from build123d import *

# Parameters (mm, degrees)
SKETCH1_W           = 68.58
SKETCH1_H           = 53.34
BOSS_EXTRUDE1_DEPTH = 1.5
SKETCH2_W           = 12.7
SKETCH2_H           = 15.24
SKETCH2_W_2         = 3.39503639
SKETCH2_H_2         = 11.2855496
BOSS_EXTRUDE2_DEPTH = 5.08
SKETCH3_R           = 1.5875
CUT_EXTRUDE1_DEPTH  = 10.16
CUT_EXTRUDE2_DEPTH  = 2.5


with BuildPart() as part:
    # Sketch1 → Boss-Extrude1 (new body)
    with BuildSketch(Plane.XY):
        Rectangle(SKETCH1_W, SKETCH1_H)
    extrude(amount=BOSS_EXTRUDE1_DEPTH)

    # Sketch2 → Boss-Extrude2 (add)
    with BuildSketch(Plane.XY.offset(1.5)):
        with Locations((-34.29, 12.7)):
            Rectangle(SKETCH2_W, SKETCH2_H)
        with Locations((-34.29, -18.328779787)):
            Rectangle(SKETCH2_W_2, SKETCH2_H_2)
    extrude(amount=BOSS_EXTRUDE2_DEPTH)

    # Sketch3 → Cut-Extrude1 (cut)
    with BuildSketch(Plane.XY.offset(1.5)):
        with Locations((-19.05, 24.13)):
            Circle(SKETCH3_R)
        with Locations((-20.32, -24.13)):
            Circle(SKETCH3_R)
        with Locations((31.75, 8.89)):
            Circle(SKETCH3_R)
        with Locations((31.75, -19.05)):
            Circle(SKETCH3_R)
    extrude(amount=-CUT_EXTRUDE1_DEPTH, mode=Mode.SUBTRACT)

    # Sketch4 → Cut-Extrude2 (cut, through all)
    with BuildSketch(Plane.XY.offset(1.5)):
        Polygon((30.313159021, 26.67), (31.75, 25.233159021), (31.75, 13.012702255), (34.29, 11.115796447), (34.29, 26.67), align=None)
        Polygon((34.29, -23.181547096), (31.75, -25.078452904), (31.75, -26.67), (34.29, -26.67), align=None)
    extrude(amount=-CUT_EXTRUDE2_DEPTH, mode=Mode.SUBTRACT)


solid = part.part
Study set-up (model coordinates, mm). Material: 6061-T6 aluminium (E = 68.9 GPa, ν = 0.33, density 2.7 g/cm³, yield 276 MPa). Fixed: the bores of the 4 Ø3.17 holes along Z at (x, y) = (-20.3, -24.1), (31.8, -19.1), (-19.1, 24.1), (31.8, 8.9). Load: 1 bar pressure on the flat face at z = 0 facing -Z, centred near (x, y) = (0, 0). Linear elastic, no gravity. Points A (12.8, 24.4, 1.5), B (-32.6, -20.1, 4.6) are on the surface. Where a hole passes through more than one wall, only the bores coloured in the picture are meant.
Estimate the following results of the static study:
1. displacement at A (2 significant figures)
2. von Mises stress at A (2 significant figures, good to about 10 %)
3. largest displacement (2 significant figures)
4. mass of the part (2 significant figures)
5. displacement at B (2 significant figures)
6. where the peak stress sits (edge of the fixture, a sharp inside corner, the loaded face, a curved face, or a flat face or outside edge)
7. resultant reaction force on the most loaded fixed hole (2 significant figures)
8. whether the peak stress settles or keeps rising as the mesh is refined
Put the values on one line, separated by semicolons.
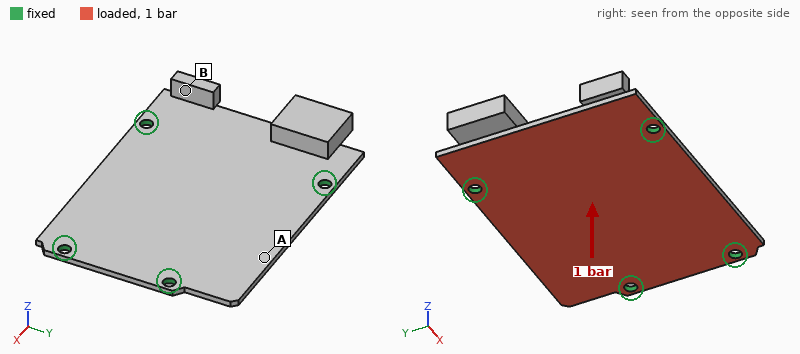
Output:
0.14 mm; 33 MPa; 0.15 mm; 18 g; 0.034 mm; edge of the fixture; 110 N; keeps rising
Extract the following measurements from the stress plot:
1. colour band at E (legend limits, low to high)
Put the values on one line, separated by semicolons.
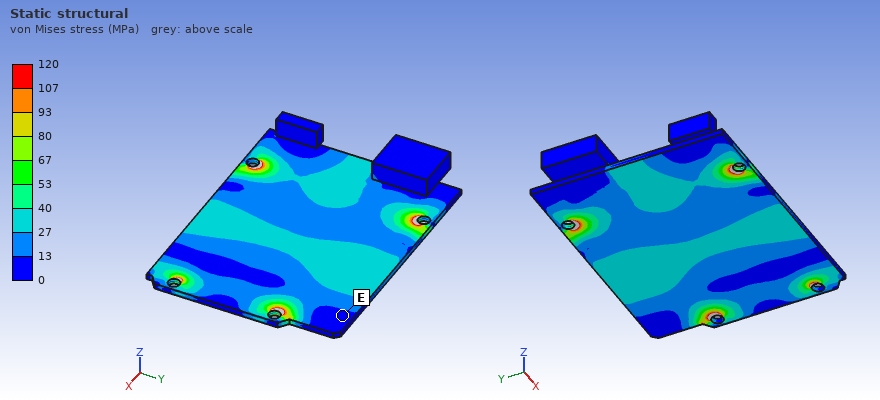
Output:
0 to 13 MPa
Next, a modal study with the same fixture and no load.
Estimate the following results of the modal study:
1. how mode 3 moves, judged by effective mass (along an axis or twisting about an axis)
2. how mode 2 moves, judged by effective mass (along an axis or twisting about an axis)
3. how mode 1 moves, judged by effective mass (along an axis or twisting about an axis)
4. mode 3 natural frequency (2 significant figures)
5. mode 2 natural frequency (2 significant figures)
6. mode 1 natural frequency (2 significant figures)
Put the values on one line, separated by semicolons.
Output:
twisting about X; along Z; along Z; 2900 Hz; 2400 Hz; 1600 Hz
